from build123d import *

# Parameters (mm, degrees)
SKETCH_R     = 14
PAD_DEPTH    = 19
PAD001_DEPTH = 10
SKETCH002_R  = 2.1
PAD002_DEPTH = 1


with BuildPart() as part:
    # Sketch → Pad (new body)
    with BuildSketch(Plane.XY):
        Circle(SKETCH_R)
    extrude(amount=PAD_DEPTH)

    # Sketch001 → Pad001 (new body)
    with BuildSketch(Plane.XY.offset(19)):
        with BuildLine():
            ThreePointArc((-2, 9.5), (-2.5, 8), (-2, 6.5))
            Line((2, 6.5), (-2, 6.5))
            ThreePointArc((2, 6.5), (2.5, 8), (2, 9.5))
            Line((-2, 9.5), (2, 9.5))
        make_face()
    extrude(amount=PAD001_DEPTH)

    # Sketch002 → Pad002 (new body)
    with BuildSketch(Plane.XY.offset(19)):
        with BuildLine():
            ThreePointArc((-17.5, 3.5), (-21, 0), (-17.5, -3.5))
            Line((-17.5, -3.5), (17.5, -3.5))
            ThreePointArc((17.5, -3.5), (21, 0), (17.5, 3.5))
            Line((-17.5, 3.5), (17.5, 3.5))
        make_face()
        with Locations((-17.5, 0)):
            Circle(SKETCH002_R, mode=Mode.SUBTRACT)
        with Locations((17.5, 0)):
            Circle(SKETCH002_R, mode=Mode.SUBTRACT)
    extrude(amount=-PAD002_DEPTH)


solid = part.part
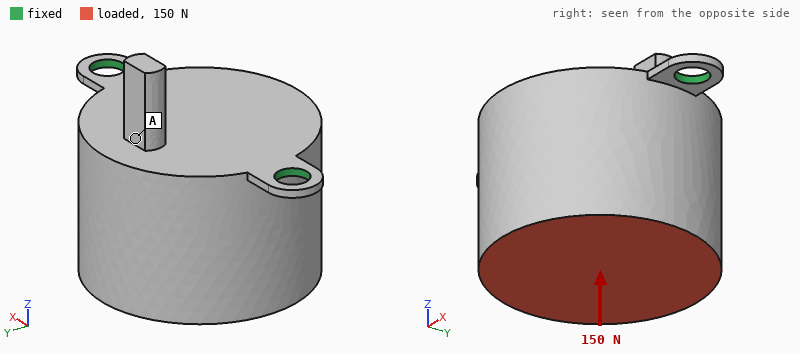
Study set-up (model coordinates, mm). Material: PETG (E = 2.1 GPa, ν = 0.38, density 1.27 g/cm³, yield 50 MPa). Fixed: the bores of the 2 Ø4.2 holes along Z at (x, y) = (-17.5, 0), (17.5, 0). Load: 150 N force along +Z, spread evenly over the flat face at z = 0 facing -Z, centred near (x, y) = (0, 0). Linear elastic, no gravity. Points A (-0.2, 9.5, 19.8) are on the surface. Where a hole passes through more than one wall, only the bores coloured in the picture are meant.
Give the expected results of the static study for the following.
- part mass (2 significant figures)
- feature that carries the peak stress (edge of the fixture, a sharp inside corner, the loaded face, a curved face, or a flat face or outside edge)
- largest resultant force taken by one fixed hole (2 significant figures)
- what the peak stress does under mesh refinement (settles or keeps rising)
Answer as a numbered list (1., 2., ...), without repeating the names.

1. 15 g
2. edge of the fixture
3. 87 N
4. keeps rising
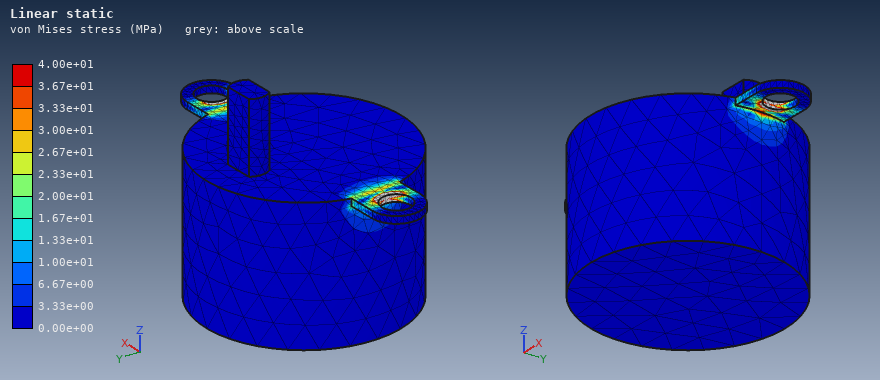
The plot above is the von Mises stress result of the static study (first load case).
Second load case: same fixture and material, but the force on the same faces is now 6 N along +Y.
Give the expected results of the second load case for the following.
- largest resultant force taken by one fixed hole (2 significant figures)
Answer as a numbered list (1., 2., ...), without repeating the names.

1. 3.0 N
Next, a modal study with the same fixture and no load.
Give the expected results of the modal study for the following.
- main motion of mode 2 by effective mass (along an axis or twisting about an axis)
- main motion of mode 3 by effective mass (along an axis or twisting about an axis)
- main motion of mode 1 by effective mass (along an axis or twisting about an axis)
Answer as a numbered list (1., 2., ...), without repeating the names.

1. along Z
2. along X
3. along Y
